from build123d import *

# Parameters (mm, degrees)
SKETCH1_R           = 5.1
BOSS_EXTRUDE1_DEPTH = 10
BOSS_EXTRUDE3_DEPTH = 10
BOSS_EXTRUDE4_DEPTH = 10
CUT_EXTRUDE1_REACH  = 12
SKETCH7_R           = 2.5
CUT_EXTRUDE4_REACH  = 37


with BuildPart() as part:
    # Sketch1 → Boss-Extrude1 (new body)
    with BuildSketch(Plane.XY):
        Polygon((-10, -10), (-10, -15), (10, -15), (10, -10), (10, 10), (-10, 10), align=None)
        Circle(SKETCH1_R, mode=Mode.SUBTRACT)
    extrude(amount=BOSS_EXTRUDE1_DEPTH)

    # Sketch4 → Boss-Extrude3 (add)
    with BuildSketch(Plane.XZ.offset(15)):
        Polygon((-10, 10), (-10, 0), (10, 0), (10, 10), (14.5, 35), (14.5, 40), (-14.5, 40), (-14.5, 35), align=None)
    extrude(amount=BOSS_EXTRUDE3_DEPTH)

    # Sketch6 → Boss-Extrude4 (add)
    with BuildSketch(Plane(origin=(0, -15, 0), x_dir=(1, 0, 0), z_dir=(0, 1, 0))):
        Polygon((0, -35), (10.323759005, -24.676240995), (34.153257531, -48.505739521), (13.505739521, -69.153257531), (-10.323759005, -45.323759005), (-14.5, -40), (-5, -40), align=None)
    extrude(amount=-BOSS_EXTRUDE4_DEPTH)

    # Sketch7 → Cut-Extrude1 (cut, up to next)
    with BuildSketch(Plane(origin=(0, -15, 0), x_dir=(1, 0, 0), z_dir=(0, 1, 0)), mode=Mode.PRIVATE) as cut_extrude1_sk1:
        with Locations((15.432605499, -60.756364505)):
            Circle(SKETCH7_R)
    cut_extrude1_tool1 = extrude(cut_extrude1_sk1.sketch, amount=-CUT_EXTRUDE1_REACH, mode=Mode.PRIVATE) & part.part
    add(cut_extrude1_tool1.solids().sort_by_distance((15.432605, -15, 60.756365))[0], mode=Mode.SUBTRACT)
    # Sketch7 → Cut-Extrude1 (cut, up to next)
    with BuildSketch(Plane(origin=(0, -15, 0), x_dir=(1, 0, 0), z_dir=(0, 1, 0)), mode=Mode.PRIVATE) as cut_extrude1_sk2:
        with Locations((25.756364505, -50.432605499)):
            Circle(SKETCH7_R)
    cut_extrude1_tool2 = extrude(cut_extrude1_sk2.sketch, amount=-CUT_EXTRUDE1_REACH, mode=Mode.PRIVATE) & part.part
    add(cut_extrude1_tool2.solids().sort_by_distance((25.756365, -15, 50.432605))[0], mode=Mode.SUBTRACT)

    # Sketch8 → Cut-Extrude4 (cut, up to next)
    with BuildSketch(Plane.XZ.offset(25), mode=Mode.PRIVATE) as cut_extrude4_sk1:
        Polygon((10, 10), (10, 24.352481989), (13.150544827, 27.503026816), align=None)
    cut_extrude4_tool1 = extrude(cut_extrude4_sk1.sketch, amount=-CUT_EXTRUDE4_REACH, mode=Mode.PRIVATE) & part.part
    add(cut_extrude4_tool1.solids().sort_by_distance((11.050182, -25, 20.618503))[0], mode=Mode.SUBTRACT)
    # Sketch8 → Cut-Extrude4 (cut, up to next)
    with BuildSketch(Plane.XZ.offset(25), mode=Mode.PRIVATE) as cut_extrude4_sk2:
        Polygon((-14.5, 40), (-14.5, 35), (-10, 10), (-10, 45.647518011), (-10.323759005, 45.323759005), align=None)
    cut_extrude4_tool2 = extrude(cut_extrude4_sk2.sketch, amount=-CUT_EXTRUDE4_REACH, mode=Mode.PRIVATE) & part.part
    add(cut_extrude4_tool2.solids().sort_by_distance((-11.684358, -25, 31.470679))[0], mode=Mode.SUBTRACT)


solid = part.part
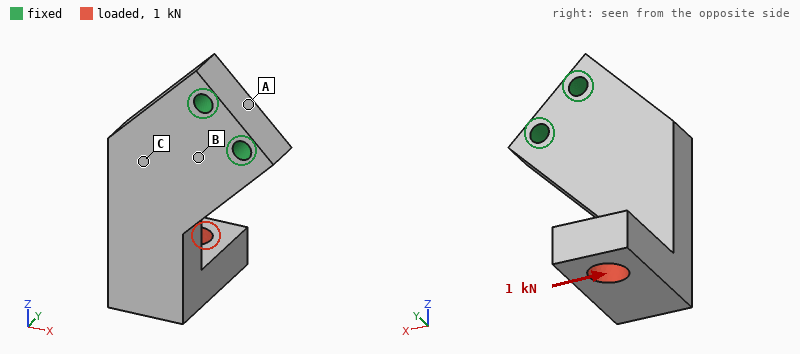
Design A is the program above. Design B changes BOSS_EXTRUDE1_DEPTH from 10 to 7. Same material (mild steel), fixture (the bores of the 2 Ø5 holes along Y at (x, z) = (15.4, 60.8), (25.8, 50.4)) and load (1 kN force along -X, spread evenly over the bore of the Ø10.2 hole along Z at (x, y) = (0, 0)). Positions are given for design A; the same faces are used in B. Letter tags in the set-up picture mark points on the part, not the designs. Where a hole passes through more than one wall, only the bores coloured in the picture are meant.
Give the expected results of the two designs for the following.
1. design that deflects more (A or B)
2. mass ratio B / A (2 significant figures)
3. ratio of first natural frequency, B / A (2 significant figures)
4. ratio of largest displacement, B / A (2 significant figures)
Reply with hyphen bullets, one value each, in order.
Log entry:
- B
- 0.94
- 1.1
- 1.1
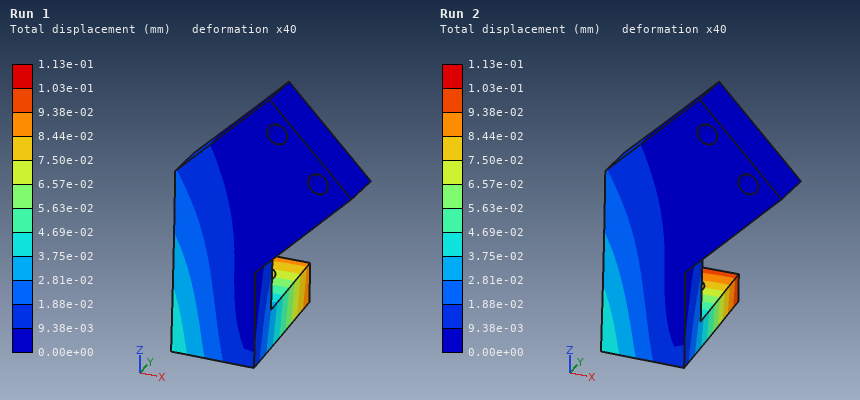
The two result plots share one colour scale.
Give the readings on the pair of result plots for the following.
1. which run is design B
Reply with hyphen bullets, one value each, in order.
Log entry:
- Run 2
